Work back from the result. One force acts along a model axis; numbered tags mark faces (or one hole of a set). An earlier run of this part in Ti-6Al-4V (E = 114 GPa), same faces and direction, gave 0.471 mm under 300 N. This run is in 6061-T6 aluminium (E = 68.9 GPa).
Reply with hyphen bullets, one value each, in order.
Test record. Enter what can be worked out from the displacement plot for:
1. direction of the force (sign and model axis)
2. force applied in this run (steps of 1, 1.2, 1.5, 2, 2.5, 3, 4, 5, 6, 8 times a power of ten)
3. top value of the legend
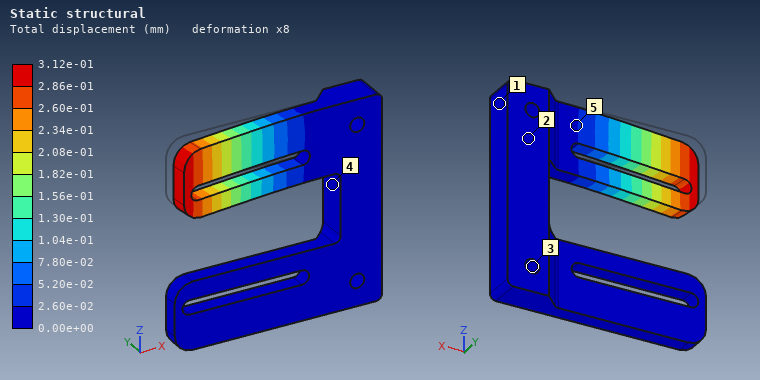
- -Y
- 120 N
- 3.12e-01 mm
